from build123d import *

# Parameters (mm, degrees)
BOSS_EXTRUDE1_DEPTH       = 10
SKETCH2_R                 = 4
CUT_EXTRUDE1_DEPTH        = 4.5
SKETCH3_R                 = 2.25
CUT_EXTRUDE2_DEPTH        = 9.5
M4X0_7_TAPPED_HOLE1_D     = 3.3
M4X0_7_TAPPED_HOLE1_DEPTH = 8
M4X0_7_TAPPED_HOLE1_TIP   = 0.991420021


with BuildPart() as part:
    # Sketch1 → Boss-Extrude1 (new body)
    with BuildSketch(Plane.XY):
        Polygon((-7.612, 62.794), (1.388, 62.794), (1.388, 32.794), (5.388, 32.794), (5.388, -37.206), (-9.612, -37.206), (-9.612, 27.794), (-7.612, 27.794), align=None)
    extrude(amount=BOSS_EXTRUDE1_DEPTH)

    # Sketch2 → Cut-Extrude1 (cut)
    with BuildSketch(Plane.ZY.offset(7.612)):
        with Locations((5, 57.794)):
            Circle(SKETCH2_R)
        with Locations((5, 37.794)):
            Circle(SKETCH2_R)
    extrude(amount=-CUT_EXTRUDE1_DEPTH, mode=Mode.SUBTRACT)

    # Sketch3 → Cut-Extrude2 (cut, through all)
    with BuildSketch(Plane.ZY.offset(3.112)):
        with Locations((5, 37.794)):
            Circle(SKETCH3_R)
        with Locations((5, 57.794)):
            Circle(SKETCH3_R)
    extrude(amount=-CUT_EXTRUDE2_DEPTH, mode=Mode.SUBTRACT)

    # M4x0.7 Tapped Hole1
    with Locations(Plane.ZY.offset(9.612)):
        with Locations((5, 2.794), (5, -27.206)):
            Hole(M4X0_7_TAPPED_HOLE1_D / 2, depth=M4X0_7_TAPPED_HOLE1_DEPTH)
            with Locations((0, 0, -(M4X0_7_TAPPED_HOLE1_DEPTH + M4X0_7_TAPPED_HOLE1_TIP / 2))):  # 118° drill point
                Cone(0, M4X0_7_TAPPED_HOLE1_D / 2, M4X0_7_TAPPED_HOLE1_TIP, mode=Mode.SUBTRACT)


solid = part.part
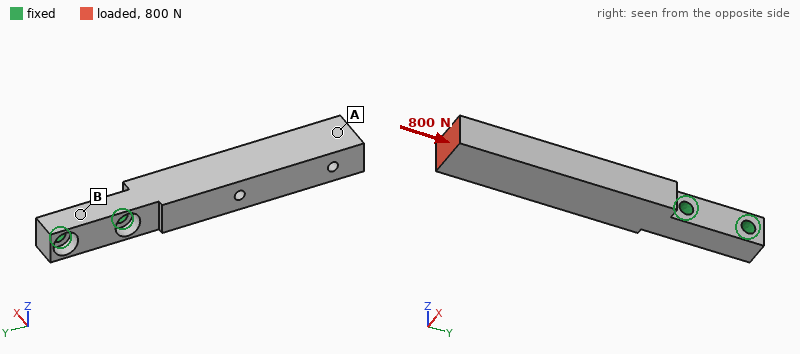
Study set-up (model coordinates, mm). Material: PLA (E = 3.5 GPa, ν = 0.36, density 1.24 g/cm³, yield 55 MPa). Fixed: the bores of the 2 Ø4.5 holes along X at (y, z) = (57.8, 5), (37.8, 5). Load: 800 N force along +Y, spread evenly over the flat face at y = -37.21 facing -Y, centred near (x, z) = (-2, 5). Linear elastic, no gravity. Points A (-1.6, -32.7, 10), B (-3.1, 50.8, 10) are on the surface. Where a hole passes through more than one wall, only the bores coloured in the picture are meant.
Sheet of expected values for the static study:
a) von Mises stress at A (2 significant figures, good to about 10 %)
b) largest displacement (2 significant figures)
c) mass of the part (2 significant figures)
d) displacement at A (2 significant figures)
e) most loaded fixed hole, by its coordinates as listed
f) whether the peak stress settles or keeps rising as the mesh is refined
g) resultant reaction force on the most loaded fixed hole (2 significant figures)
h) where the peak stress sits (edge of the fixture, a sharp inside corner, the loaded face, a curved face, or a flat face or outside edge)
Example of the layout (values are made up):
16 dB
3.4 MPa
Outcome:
5.8 MPa
0.37 mm
15 g
0.32 mm
(37.8, 5)
keeps rising
720 N
edge of the fixture
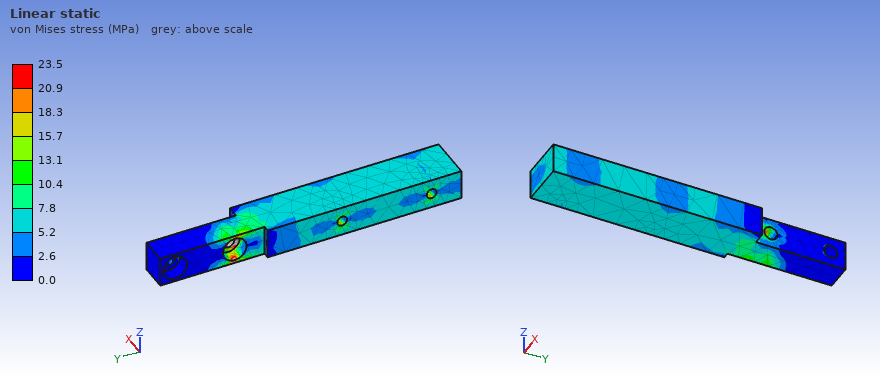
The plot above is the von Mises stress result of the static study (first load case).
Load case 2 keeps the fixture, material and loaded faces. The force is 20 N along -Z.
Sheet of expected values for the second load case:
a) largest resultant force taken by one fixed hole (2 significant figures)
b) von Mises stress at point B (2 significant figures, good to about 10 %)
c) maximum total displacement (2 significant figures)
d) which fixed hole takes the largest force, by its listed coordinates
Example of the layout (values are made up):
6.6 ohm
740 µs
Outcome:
52 N
1.3 MPa
0.98 mm
(37.8, 5)
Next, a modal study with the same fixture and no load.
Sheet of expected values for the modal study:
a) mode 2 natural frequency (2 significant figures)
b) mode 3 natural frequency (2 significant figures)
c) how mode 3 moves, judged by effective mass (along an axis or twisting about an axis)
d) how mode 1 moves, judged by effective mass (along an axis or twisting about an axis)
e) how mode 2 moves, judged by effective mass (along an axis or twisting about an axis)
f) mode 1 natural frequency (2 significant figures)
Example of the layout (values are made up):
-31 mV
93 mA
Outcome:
380 Hz
2300 Hz
twisting about Y
along X
along Z
350 Hz
